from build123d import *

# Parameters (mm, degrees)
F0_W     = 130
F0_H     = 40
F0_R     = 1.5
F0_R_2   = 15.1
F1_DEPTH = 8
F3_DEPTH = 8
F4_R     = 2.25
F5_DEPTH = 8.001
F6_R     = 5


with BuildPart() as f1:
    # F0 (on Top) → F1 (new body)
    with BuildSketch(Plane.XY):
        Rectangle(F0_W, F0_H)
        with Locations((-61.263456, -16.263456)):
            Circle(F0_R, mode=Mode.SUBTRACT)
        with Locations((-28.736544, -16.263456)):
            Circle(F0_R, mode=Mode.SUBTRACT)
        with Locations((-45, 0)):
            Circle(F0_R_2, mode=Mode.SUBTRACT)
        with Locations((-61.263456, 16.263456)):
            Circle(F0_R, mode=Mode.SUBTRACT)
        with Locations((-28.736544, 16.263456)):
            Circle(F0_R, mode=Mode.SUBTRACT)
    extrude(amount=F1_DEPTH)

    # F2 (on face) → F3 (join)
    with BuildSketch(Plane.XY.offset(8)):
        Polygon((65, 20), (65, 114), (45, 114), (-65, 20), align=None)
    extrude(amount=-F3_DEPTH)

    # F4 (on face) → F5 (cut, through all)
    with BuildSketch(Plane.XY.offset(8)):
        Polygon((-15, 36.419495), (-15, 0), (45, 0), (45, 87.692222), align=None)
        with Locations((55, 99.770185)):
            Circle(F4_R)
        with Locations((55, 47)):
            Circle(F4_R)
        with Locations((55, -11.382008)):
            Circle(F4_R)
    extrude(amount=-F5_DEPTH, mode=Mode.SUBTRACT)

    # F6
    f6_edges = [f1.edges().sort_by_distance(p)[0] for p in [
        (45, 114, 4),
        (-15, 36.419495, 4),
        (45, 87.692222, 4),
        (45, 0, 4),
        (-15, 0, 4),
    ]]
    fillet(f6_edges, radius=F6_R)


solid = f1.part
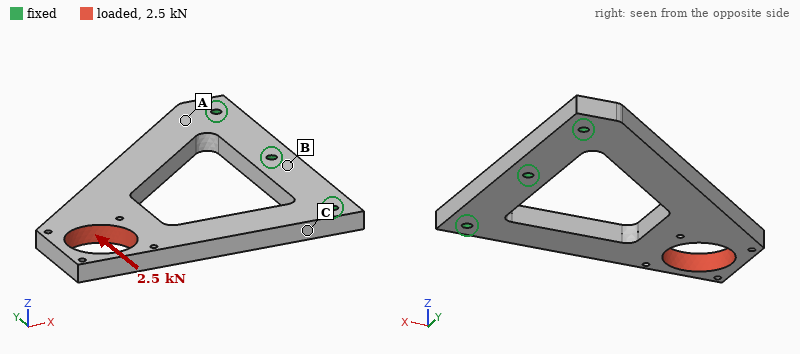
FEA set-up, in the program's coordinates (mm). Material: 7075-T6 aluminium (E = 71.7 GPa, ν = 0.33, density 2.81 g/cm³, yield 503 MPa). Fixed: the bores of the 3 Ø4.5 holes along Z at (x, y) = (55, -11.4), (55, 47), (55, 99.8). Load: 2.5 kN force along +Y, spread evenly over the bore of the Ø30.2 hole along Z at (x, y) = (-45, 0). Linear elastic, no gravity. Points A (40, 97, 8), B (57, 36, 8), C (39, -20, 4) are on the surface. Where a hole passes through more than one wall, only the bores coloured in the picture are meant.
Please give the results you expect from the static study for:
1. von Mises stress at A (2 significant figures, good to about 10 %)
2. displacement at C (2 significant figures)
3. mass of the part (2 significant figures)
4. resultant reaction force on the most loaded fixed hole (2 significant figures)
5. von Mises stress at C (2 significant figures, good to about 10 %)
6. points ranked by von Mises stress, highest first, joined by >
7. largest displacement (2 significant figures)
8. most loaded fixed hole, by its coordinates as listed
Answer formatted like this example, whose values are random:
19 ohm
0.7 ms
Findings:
21 MPa
0.018 mm
170 g
2.7 kN
35 MPa
C > A > B
0.11 mm
(55, 99.8)
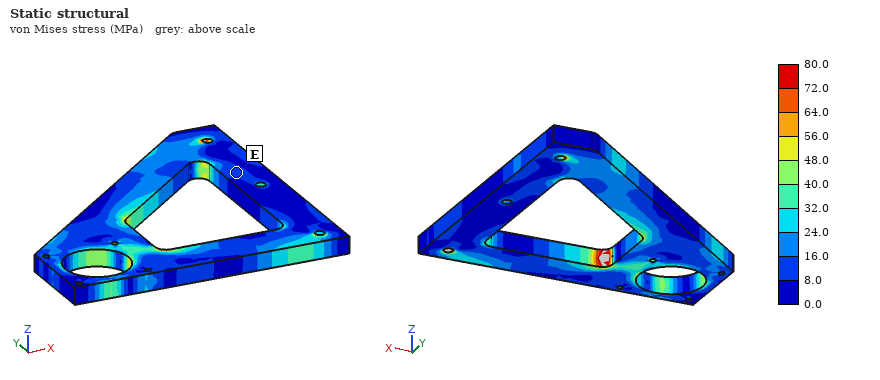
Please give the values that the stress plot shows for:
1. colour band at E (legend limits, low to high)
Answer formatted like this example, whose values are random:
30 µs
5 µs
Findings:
8.0 to 16.0 MPa
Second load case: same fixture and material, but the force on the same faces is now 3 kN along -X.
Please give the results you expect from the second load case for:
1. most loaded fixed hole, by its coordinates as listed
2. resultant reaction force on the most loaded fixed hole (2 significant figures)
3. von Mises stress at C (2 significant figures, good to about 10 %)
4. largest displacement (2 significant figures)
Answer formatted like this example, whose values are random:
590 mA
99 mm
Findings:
(55, -11.4)
2.6 kN
22 MPa
53 µm
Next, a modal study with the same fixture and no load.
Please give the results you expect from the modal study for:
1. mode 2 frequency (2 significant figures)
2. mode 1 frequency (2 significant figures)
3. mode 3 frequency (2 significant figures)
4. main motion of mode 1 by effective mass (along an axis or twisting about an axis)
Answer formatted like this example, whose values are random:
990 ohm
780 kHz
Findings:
1600 Hz
440 Hz
2500 Hz
along Z
